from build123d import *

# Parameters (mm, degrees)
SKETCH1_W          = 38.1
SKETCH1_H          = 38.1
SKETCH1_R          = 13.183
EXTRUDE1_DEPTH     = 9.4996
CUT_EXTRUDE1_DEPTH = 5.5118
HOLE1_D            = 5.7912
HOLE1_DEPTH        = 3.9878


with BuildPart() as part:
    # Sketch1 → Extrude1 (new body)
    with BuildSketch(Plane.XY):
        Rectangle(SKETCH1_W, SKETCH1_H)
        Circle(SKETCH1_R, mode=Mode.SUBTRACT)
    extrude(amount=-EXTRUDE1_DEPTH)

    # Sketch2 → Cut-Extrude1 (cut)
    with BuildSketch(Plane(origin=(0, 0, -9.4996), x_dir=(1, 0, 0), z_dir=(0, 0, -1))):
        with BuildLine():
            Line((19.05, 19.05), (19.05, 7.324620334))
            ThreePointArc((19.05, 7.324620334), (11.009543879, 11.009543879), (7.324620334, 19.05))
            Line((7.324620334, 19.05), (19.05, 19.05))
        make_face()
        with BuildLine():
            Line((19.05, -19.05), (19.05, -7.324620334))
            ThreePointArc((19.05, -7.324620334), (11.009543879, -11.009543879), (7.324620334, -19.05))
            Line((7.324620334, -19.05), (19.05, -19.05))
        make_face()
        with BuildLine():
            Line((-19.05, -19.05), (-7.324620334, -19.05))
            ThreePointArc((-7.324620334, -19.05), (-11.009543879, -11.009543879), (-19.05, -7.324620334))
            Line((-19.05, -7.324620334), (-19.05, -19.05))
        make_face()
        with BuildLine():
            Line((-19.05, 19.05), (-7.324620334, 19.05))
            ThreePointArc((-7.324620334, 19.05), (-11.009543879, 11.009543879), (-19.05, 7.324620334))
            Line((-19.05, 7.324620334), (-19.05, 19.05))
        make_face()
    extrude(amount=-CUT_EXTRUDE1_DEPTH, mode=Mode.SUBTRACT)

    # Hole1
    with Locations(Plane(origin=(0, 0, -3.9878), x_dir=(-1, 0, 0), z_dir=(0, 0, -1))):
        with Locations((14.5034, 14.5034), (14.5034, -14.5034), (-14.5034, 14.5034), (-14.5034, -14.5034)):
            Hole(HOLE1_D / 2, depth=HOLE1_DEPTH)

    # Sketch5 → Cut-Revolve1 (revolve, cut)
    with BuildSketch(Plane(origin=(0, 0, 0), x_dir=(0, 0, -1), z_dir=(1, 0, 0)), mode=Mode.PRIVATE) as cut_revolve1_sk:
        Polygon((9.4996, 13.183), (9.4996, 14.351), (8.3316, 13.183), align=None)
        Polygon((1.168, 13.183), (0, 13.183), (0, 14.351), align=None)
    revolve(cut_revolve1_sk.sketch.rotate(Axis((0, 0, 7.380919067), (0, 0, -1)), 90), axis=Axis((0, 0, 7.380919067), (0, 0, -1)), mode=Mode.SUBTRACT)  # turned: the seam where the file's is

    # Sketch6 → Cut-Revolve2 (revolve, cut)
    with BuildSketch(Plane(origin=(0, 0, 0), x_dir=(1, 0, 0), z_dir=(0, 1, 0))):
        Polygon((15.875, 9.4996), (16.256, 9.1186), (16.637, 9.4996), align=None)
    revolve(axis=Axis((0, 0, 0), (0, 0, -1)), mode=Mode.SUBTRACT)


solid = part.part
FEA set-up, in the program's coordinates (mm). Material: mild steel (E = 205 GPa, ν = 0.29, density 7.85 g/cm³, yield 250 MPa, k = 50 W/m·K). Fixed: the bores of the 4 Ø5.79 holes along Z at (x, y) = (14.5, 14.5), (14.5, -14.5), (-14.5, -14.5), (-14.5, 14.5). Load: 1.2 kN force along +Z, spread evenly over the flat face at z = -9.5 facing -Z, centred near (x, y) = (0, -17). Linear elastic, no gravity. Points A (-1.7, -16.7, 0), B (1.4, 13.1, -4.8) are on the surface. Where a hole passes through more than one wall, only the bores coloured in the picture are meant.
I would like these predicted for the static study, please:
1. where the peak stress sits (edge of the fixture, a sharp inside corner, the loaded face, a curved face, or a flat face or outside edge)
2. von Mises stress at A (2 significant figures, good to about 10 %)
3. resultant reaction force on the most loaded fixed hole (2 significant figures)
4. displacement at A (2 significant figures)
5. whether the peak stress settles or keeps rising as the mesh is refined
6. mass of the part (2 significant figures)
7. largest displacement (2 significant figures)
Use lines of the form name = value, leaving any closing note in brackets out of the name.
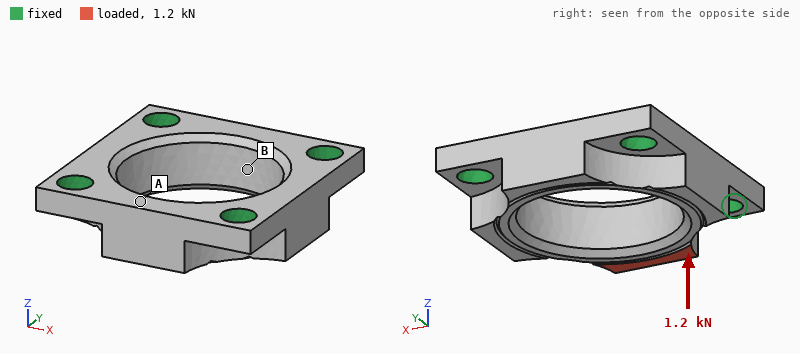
where the peak stress sits = edge of the fixture
von Mises stress at A = 22 MPa
resultant reaction force on the most loaded fixed hole = 690 N
displacement at A = 4.3 µm
whether the peak stress settles or keeps rising as the mesh is refined = keeps rising
mass of the part = 45 g
largest displacement = 6.7 µm
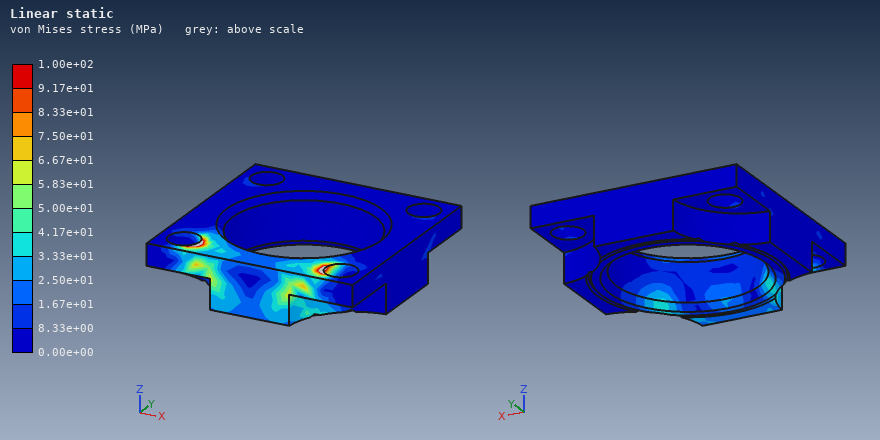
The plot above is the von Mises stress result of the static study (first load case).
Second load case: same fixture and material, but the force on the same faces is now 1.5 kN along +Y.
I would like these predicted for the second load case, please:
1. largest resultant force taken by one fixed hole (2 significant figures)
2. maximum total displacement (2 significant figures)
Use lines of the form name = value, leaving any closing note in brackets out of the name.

largest resultant force taken by one fixed hole = 700 N
maximum total displacement = 12 µm
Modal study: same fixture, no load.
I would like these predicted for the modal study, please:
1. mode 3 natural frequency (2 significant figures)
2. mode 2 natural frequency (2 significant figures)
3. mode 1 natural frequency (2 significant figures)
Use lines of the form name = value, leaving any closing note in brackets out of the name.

mode 3 natural frequency = 32 kHz
mode 2 natural frequency = 32 kHz
mode 1 natural frequency = 26 kHz
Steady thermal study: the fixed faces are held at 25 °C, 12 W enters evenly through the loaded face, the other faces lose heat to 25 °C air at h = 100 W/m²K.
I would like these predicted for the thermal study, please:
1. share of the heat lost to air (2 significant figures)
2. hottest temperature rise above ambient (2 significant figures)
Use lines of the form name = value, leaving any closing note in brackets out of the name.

share of the heat lost to air = 12 %
hottest temperature rise above ambient = 36 K
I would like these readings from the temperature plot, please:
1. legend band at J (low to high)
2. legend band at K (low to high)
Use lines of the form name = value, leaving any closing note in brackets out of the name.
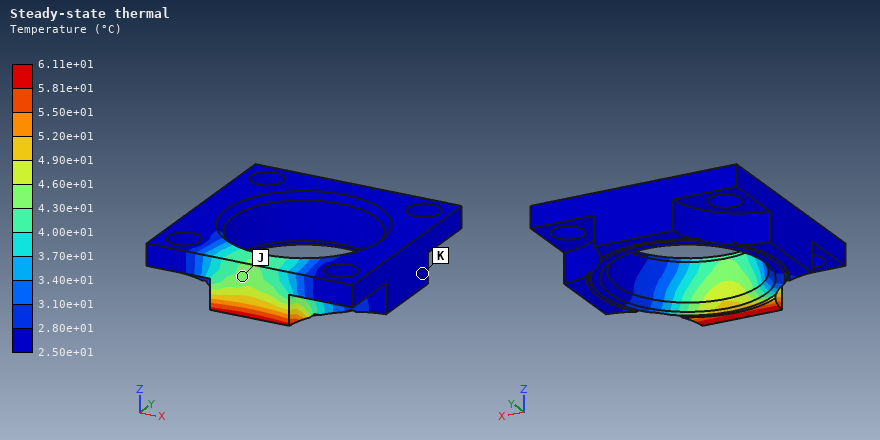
legend band at J = 4.30e+01 to 4.60e+01 °C
legend band at K = 2.50e+01 to 2.80e+01 °C
